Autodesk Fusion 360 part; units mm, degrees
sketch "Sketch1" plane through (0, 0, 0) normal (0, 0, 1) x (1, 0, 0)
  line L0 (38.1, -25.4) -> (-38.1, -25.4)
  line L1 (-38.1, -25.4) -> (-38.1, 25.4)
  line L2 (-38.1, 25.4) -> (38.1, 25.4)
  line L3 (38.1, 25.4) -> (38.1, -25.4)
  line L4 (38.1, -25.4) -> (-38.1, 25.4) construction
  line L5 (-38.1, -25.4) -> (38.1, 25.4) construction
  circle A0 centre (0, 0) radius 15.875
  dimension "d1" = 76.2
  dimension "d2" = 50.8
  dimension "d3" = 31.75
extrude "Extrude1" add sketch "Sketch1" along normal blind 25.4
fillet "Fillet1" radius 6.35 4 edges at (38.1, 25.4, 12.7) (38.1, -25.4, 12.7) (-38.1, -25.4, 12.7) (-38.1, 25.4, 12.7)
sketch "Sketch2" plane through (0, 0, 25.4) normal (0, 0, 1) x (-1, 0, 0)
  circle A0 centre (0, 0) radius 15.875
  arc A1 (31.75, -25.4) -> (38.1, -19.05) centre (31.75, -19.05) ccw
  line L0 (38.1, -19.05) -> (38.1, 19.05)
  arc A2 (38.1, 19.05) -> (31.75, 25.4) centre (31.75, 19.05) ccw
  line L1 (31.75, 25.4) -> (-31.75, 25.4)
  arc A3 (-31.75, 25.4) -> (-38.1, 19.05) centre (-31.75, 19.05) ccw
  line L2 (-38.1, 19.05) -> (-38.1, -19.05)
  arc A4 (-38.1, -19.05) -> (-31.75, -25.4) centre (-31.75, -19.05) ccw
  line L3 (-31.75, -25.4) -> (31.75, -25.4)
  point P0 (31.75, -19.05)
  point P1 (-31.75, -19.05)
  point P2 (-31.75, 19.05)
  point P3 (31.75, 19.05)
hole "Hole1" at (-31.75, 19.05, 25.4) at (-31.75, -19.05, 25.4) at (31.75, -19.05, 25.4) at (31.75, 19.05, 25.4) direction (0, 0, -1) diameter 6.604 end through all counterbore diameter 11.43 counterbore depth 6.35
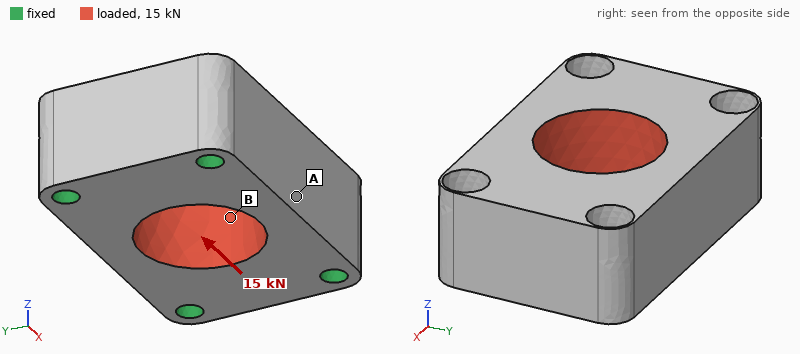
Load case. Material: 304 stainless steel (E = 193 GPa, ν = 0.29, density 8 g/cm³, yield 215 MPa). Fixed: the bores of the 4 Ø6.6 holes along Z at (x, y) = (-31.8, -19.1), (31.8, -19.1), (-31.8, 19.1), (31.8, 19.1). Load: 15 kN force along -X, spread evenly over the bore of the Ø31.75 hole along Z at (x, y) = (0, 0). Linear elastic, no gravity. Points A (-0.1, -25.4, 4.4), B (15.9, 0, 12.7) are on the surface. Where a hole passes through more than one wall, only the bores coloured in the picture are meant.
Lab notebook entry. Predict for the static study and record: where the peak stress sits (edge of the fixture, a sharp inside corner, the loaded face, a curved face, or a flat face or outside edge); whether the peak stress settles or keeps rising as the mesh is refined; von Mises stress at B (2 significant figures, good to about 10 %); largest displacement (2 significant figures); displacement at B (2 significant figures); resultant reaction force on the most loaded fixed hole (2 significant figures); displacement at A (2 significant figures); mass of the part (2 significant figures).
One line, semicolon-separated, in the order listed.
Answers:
edge of the fixture; keeps rising; 6.0 MPa; 1.6 µm; 1.2 µm; 3.9 kN; 0.88 µm; 580 g
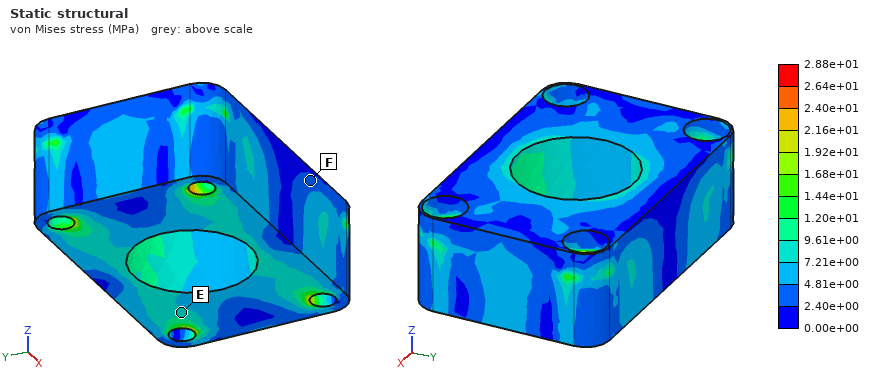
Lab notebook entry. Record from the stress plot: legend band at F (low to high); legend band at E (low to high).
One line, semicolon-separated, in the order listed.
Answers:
2.40e+00 to 4.81e+00 MPa; 7.21e+00 to 9.61e+00 MPa
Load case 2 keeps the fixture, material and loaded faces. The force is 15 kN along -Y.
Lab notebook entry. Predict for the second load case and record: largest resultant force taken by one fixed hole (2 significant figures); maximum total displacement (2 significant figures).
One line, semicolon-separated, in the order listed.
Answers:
4.3 kN; 4.0 µm
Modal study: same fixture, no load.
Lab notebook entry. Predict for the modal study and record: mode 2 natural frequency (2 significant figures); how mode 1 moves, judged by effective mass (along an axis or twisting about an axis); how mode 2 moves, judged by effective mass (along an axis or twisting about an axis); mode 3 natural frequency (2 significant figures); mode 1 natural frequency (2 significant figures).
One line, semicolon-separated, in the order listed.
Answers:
20 kHz; along Z; twisting about X; 21 kHz; 17 kHz
